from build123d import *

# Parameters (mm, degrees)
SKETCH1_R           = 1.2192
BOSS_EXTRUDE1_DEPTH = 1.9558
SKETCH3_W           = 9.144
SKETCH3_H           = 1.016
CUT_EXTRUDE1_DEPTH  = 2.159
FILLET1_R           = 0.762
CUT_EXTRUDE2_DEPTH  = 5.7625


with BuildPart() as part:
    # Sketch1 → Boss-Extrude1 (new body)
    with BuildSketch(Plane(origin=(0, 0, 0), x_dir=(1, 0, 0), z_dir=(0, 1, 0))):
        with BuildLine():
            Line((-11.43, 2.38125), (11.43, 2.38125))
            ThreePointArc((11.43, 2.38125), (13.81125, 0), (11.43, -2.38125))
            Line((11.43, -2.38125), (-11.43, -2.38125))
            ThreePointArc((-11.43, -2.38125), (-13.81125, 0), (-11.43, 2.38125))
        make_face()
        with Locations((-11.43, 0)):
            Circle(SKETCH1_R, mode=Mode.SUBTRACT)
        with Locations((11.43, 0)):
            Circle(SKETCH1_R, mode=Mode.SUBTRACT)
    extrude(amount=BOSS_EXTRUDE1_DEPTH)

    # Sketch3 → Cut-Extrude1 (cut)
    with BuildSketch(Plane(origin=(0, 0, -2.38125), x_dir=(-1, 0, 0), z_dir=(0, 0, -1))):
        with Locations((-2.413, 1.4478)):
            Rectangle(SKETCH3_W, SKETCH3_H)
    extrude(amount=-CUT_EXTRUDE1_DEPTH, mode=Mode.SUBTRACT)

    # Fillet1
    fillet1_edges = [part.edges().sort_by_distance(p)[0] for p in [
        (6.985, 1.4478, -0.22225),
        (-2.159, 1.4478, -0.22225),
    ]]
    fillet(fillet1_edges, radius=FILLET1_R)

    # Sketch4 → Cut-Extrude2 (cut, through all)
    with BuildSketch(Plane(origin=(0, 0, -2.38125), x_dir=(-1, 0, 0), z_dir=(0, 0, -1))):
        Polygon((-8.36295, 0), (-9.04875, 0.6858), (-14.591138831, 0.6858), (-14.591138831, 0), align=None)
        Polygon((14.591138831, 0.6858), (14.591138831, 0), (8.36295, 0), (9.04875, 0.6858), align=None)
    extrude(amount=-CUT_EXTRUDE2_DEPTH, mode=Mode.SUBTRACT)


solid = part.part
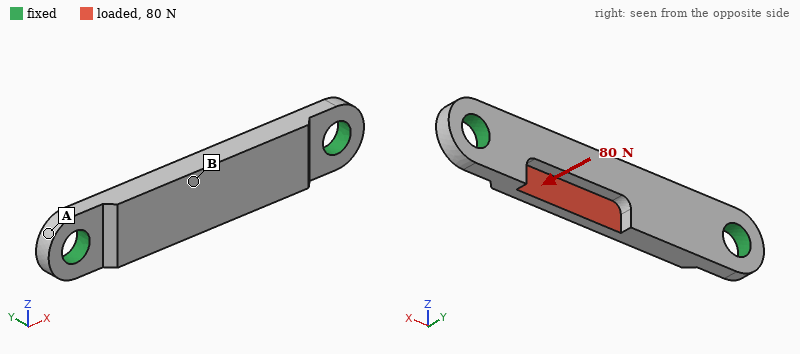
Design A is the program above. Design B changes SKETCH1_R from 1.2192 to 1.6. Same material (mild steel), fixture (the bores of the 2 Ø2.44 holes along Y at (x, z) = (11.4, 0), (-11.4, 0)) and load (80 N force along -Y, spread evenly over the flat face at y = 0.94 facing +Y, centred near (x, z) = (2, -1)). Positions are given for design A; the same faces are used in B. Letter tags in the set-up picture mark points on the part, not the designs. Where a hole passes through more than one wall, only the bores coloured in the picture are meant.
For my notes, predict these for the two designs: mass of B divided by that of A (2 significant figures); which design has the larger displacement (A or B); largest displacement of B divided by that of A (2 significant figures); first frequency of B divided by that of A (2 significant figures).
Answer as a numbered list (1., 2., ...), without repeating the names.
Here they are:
1. 0.95
2. A
3. 0.88
4. 1.1
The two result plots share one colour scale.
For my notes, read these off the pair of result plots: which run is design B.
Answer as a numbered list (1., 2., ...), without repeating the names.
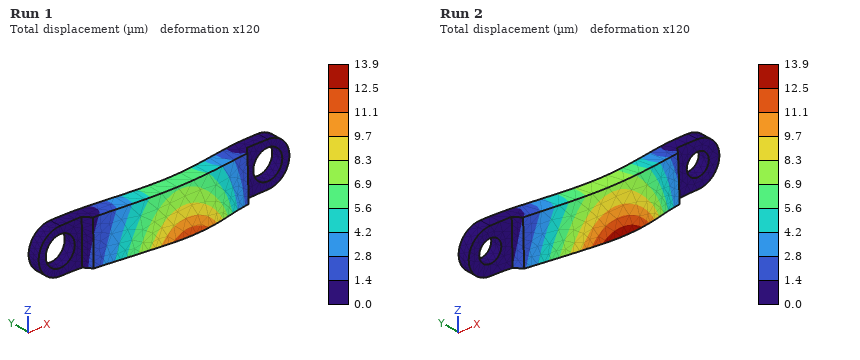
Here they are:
1. Run 1
